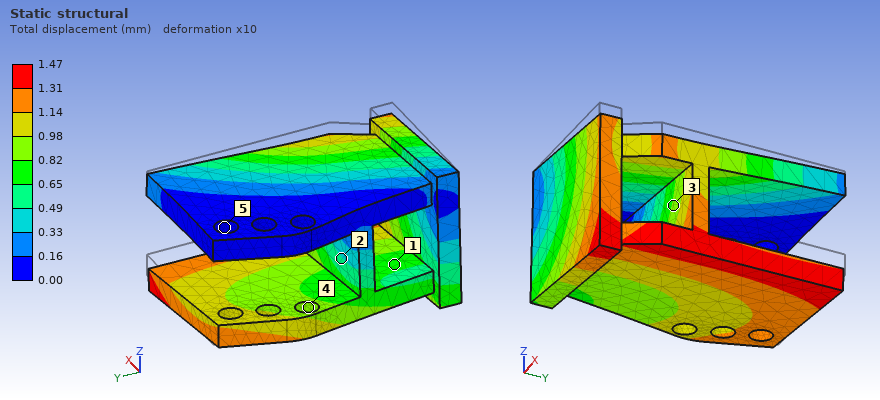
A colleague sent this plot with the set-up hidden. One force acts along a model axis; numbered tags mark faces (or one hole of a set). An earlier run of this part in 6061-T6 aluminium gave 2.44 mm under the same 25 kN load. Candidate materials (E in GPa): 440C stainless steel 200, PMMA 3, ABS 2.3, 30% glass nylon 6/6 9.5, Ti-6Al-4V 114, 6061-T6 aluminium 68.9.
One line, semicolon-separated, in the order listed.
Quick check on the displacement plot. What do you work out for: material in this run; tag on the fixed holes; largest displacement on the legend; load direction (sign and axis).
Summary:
Ti-6Al-4V; 5; 1.47 mm; -X
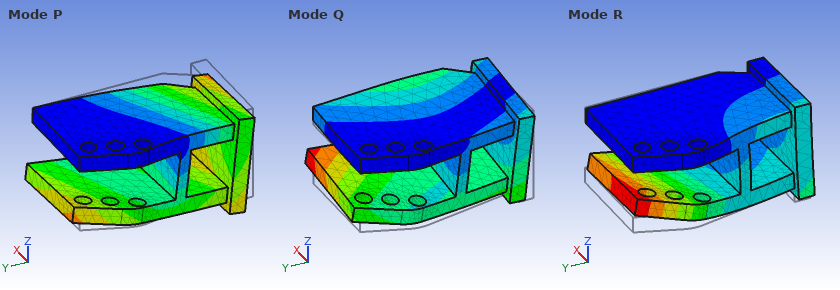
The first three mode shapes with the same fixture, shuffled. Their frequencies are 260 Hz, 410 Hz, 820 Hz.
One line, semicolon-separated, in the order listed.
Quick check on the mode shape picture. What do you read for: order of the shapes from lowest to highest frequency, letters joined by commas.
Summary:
P, Q, R
